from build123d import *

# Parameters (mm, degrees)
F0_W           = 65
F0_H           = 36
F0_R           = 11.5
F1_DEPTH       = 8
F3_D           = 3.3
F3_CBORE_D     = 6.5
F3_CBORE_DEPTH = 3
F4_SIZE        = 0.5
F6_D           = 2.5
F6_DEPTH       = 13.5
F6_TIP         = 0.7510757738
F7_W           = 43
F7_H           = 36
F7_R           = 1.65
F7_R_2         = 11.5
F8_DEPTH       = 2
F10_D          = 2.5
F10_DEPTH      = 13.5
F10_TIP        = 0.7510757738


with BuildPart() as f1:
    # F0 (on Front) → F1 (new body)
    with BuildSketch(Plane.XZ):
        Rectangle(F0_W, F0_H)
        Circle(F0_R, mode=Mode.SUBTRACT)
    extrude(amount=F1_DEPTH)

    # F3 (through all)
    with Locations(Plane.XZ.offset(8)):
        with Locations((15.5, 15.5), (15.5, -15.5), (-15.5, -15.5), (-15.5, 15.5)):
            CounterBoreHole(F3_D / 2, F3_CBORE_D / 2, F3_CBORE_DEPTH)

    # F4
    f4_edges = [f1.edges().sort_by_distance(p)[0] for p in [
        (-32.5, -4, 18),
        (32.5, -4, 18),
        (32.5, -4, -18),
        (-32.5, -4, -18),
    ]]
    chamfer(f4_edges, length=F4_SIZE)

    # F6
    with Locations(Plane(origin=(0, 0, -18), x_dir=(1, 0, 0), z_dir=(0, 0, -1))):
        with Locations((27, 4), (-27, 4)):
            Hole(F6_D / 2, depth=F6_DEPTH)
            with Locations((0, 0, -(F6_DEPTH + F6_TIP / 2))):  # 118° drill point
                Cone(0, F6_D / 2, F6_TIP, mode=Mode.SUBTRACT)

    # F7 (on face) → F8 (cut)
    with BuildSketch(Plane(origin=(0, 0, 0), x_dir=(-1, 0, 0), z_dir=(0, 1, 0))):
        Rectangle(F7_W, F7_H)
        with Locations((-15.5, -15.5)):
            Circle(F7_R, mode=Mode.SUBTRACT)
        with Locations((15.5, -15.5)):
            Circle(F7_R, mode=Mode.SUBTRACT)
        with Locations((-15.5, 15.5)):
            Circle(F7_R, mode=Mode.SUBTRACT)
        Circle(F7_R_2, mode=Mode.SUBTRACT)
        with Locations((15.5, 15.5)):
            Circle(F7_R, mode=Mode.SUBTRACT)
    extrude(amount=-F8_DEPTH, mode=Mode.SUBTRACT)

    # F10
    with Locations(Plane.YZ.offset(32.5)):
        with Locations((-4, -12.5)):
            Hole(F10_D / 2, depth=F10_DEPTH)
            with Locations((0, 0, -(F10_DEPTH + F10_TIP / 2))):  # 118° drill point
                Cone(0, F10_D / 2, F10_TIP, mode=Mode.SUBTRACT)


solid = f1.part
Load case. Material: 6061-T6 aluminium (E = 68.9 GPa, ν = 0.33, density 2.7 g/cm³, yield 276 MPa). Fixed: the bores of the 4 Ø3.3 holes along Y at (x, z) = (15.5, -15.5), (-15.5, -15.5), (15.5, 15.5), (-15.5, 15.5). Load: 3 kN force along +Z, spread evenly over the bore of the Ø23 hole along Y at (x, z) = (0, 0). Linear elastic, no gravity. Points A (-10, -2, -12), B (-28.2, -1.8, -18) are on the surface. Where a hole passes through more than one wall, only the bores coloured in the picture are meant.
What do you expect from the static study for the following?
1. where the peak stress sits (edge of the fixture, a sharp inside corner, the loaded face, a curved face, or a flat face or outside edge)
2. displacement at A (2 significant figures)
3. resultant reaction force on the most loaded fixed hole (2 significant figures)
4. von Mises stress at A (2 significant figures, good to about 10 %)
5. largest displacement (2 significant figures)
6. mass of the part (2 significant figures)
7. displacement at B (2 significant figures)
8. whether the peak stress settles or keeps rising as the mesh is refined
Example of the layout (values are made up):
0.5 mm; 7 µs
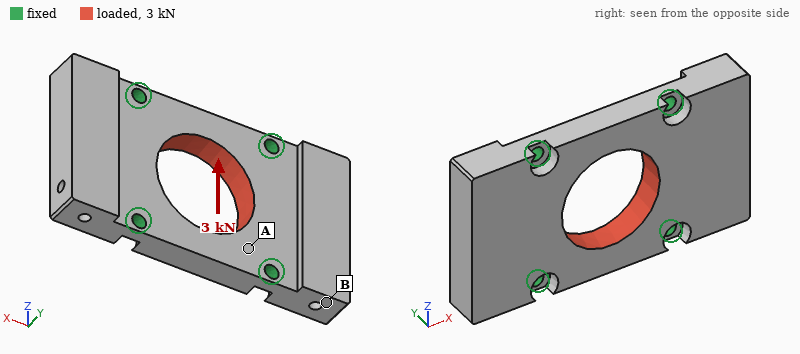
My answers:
edge of the fixture; 3.3 µm; 780 N; 15 MPa; 8.4 µm; 34 g; 1.6 µm; keeps rising
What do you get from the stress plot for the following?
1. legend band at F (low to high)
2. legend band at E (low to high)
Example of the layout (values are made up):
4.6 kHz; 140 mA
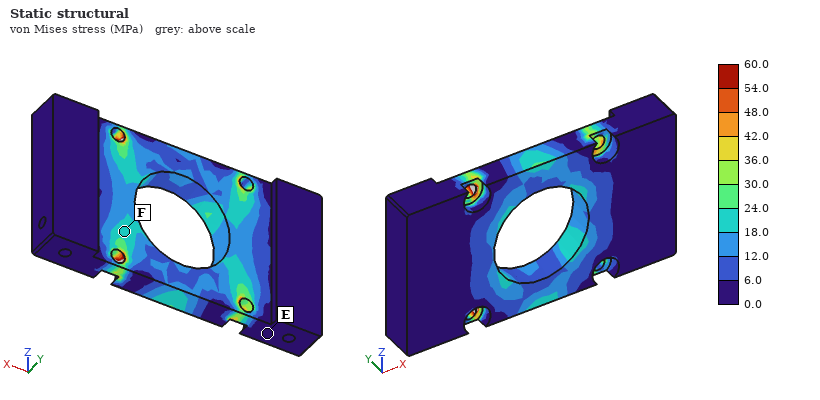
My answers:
18.0 to 24.0 MPa; 0.0 to 6.0 MPa
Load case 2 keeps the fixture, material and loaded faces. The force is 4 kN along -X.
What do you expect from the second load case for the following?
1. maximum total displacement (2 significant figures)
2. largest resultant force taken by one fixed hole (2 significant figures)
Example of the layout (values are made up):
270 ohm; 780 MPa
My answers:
9.4 µm; 1.0 kN
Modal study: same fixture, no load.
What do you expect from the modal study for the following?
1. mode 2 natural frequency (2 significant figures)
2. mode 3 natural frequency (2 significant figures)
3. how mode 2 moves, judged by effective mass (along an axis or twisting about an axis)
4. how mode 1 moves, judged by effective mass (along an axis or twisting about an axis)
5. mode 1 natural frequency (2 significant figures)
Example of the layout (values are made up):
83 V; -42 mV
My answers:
7600 Hz; 18 kHz; twisting about Z; along Y; 7100 Hz
